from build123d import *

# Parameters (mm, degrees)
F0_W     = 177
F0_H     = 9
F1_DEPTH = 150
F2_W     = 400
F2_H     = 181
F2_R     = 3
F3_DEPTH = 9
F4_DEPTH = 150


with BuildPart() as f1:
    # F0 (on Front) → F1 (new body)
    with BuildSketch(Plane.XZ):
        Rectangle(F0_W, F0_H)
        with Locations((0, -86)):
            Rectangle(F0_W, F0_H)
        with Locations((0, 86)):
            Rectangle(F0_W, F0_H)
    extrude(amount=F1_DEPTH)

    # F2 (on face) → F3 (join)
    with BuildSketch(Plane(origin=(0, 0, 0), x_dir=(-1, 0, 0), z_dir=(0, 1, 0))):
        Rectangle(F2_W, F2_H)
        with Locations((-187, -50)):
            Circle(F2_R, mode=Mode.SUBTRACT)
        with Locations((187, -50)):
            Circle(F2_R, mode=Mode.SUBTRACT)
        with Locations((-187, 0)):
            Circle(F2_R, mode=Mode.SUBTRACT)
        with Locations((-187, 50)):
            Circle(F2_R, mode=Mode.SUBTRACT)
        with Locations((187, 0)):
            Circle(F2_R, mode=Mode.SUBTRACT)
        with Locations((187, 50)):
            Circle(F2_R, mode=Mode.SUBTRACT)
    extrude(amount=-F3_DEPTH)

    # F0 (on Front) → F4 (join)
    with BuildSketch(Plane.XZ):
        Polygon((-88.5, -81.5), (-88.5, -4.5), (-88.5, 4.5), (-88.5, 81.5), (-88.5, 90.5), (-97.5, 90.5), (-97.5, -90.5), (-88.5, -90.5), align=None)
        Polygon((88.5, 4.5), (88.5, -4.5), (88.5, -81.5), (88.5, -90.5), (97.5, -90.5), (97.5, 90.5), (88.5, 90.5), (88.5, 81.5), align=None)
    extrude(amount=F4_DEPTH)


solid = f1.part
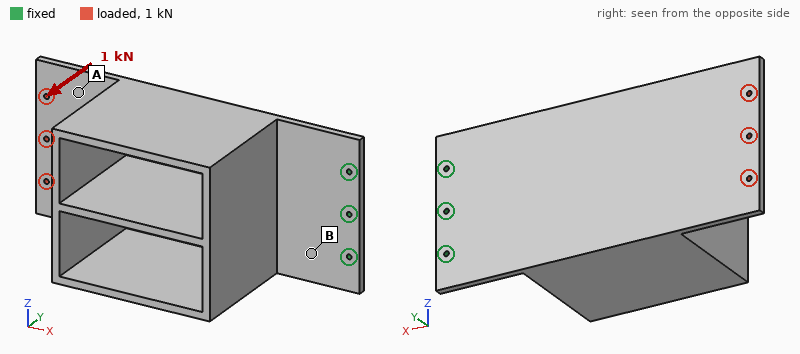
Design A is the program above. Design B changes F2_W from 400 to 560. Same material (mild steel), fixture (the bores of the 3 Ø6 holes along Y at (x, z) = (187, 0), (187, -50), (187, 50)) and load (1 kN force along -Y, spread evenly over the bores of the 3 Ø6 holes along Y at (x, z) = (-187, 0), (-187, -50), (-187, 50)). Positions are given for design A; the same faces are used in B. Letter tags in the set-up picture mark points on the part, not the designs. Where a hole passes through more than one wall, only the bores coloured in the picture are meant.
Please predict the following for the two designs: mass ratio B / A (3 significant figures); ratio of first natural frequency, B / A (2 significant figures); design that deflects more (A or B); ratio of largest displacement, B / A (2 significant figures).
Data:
1.15
0.88
B
1.2
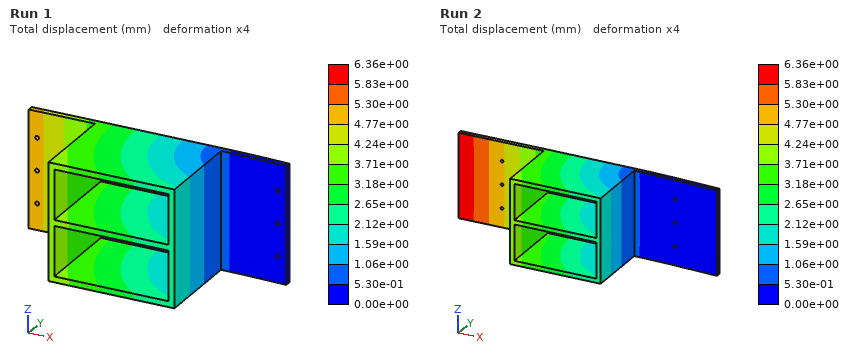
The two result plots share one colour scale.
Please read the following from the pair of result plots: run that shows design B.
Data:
Run 2
